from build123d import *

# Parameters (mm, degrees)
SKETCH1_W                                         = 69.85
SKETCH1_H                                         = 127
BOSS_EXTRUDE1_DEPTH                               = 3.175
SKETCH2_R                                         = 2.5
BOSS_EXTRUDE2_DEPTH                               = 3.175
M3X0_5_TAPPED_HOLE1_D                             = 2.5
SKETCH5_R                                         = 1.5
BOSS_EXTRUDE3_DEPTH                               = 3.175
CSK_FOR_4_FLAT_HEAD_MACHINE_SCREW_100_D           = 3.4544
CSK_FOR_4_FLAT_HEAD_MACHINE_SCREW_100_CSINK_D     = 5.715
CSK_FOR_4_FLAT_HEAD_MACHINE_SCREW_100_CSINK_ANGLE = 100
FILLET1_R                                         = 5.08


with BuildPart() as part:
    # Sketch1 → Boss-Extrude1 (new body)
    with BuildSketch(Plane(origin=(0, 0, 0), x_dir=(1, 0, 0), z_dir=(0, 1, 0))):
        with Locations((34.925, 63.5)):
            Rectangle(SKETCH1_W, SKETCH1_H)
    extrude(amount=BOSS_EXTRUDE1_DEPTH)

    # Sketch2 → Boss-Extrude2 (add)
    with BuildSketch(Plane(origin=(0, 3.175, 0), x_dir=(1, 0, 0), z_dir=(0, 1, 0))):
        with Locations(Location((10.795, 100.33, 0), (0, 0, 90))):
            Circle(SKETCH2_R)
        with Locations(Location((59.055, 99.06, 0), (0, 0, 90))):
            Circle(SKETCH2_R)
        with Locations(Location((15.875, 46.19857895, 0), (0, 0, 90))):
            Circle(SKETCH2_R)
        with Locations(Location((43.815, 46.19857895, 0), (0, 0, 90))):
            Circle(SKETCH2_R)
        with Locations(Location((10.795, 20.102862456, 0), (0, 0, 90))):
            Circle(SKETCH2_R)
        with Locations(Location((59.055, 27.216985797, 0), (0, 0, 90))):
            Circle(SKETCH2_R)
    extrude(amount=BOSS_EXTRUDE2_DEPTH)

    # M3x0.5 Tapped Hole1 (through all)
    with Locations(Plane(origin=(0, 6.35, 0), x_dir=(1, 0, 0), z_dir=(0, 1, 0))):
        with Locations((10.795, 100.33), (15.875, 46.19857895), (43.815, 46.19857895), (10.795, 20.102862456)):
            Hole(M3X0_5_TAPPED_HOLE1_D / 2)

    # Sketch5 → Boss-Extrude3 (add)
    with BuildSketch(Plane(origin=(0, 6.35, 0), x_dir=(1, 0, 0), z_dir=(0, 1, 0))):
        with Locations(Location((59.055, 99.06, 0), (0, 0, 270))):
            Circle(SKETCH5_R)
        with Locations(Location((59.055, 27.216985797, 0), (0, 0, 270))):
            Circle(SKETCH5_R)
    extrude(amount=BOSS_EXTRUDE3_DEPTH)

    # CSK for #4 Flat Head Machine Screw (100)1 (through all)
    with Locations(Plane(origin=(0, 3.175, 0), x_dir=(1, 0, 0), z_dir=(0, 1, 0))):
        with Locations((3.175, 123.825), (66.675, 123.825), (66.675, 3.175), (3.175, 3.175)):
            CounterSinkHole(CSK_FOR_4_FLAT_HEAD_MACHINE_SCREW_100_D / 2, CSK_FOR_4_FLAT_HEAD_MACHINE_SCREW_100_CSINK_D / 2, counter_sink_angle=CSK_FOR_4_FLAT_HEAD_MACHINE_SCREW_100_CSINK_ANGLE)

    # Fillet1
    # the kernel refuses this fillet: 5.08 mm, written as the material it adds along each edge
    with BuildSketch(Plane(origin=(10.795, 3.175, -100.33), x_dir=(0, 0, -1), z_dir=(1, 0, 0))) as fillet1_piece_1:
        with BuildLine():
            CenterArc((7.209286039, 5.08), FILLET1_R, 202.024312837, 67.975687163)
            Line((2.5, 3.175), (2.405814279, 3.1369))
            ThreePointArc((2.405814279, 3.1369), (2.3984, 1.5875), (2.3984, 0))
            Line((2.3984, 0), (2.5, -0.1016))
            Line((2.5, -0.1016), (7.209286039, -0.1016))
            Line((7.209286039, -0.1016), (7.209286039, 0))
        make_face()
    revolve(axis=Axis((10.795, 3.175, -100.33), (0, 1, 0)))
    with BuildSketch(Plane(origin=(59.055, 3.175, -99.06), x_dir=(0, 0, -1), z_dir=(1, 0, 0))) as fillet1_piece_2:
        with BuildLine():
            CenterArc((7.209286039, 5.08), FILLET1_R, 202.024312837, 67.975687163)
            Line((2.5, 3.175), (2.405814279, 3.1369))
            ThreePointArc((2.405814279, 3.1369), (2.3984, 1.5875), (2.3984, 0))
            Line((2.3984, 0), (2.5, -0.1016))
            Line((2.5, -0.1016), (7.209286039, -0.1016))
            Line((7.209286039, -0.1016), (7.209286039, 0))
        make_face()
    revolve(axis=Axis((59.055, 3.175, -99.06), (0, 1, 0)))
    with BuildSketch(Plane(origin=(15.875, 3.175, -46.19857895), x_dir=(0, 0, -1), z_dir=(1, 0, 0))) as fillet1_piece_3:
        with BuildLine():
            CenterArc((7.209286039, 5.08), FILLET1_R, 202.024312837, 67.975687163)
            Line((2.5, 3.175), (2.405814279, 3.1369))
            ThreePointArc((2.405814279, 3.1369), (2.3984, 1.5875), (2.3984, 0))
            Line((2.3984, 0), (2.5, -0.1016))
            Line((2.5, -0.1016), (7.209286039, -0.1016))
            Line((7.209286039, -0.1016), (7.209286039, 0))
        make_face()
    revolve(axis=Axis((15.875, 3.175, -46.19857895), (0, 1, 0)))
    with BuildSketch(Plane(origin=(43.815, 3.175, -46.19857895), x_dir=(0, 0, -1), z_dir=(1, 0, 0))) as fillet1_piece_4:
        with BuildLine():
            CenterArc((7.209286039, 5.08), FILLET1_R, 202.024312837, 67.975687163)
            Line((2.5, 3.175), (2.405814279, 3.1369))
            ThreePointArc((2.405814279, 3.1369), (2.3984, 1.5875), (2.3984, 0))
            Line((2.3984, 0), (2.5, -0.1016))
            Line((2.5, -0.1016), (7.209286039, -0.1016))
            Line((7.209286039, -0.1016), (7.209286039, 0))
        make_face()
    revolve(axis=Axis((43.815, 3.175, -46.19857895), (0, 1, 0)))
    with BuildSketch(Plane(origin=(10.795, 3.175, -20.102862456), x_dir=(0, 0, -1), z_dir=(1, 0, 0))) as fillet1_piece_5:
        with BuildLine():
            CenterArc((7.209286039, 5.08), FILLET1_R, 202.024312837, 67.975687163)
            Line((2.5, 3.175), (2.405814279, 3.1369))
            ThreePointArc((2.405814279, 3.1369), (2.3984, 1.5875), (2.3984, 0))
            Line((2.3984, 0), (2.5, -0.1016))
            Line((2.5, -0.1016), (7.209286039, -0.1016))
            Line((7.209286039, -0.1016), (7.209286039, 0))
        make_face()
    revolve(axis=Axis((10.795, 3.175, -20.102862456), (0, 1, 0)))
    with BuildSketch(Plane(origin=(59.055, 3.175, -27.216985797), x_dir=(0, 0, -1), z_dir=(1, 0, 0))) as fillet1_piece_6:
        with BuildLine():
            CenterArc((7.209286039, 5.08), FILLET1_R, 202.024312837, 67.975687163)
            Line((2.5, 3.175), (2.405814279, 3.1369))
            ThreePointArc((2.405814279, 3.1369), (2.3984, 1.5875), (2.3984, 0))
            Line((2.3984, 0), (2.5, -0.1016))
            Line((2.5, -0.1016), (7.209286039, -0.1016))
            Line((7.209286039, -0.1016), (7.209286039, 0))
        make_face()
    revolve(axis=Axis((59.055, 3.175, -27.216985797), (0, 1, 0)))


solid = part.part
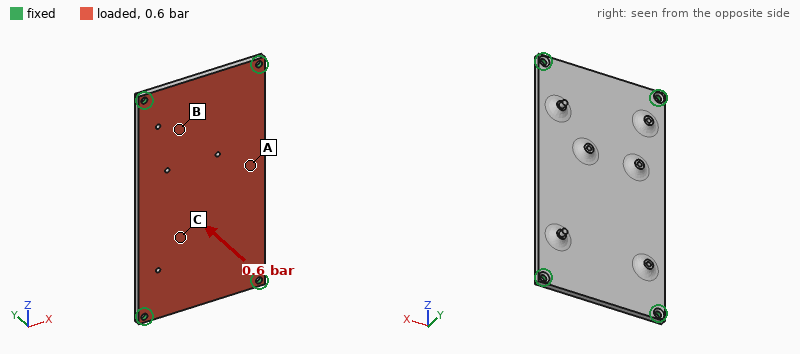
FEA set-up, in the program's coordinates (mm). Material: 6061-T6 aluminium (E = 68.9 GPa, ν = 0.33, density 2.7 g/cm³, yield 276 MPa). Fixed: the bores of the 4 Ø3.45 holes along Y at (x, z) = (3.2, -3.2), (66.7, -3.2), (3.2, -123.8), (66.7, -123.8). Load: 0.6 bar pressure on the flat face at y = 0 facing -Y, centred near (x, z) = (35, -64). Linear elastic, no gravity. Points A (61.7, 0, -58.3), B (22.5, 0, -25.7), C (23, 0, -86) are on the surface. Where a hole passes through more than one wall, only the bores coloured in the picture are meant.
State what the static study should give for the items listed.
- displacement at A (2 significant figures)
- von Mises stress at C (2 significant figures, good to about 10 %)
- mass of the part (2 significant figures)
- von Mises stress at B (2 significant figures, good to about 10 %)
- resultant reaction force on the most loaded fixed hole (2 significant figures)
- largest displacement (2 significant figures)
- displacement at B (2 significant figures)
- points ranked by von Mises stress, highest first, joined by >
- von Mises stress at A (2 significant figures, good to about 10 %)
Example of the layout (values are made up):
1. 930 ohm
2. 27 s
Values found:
1. 0.30 mm
2. 19 MPa
3. 78 g
4. 9.6 MPa
5. 160 N
6. 0.31 mm
7. 0.15 mm
8. A > C > B
9. 28 MPa
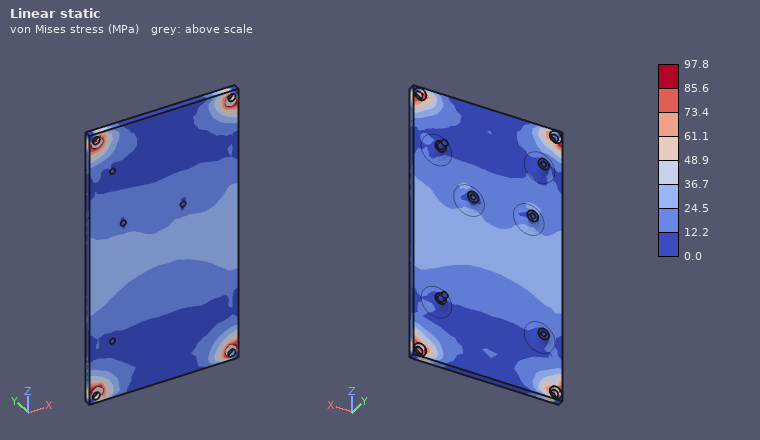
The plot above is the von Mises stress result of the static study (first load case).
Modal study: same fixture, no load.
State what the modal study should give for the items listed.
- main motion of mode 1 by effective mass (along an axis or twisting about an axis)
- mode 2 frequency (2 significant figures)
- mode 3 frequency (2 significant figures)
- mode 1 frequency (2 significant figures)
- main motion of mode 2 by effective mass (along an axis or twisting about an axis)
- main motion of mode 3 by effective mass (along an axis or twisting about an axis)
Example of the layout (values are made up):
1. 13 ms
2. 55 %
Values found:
1. along Y
2. 1700 Hz
3. 2400 Hz
4. 860 Hz
5. twisting about Z
6. twisting about X
